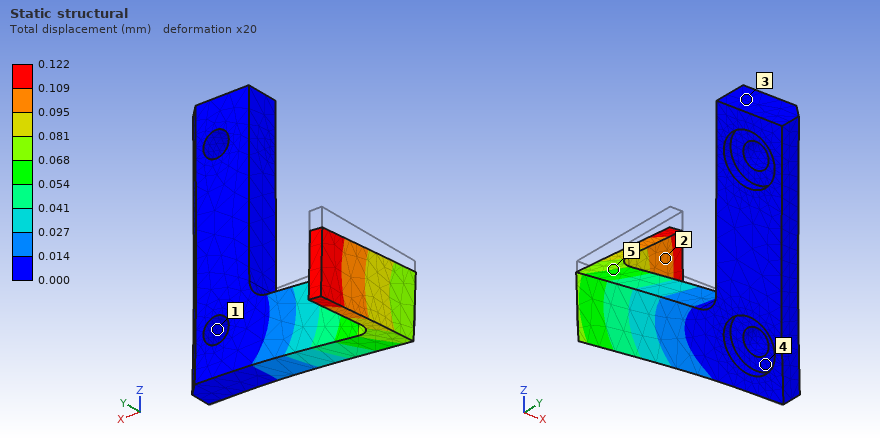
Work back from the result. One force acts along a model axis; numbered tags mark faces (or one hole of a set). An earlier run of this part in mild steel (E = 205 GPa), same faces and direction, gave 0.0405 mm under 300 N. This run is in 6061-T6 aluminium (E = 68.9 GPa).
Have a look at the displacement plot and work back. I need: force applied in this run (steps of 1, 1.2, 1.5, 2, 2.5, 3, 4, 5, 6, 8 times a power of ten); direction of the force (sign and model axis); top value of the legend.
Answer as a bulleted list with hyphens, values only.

- 300 N
- -Z
- 0.122 mm
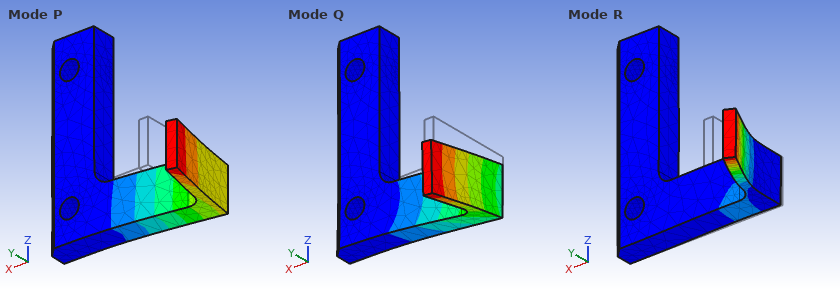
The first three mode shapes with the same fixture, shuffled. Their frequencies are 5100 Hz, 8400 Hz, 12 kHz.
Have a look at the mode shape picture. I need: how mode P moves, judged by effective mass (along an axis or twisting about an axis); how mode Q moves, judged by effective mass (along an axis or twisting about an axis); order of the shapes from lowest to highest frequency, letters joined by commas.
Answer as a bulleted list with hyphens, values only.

- along Y
- along Z
- P, Q, R
